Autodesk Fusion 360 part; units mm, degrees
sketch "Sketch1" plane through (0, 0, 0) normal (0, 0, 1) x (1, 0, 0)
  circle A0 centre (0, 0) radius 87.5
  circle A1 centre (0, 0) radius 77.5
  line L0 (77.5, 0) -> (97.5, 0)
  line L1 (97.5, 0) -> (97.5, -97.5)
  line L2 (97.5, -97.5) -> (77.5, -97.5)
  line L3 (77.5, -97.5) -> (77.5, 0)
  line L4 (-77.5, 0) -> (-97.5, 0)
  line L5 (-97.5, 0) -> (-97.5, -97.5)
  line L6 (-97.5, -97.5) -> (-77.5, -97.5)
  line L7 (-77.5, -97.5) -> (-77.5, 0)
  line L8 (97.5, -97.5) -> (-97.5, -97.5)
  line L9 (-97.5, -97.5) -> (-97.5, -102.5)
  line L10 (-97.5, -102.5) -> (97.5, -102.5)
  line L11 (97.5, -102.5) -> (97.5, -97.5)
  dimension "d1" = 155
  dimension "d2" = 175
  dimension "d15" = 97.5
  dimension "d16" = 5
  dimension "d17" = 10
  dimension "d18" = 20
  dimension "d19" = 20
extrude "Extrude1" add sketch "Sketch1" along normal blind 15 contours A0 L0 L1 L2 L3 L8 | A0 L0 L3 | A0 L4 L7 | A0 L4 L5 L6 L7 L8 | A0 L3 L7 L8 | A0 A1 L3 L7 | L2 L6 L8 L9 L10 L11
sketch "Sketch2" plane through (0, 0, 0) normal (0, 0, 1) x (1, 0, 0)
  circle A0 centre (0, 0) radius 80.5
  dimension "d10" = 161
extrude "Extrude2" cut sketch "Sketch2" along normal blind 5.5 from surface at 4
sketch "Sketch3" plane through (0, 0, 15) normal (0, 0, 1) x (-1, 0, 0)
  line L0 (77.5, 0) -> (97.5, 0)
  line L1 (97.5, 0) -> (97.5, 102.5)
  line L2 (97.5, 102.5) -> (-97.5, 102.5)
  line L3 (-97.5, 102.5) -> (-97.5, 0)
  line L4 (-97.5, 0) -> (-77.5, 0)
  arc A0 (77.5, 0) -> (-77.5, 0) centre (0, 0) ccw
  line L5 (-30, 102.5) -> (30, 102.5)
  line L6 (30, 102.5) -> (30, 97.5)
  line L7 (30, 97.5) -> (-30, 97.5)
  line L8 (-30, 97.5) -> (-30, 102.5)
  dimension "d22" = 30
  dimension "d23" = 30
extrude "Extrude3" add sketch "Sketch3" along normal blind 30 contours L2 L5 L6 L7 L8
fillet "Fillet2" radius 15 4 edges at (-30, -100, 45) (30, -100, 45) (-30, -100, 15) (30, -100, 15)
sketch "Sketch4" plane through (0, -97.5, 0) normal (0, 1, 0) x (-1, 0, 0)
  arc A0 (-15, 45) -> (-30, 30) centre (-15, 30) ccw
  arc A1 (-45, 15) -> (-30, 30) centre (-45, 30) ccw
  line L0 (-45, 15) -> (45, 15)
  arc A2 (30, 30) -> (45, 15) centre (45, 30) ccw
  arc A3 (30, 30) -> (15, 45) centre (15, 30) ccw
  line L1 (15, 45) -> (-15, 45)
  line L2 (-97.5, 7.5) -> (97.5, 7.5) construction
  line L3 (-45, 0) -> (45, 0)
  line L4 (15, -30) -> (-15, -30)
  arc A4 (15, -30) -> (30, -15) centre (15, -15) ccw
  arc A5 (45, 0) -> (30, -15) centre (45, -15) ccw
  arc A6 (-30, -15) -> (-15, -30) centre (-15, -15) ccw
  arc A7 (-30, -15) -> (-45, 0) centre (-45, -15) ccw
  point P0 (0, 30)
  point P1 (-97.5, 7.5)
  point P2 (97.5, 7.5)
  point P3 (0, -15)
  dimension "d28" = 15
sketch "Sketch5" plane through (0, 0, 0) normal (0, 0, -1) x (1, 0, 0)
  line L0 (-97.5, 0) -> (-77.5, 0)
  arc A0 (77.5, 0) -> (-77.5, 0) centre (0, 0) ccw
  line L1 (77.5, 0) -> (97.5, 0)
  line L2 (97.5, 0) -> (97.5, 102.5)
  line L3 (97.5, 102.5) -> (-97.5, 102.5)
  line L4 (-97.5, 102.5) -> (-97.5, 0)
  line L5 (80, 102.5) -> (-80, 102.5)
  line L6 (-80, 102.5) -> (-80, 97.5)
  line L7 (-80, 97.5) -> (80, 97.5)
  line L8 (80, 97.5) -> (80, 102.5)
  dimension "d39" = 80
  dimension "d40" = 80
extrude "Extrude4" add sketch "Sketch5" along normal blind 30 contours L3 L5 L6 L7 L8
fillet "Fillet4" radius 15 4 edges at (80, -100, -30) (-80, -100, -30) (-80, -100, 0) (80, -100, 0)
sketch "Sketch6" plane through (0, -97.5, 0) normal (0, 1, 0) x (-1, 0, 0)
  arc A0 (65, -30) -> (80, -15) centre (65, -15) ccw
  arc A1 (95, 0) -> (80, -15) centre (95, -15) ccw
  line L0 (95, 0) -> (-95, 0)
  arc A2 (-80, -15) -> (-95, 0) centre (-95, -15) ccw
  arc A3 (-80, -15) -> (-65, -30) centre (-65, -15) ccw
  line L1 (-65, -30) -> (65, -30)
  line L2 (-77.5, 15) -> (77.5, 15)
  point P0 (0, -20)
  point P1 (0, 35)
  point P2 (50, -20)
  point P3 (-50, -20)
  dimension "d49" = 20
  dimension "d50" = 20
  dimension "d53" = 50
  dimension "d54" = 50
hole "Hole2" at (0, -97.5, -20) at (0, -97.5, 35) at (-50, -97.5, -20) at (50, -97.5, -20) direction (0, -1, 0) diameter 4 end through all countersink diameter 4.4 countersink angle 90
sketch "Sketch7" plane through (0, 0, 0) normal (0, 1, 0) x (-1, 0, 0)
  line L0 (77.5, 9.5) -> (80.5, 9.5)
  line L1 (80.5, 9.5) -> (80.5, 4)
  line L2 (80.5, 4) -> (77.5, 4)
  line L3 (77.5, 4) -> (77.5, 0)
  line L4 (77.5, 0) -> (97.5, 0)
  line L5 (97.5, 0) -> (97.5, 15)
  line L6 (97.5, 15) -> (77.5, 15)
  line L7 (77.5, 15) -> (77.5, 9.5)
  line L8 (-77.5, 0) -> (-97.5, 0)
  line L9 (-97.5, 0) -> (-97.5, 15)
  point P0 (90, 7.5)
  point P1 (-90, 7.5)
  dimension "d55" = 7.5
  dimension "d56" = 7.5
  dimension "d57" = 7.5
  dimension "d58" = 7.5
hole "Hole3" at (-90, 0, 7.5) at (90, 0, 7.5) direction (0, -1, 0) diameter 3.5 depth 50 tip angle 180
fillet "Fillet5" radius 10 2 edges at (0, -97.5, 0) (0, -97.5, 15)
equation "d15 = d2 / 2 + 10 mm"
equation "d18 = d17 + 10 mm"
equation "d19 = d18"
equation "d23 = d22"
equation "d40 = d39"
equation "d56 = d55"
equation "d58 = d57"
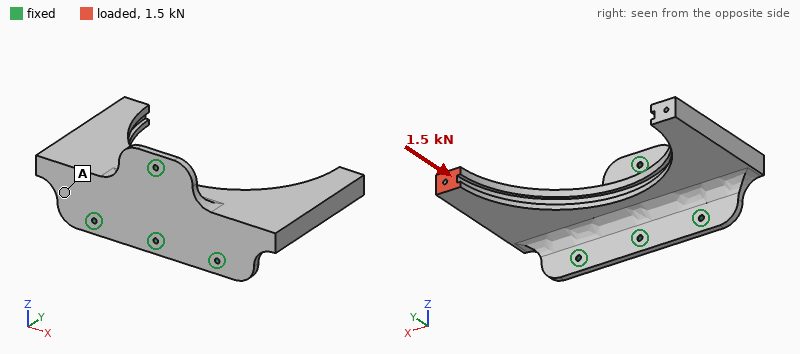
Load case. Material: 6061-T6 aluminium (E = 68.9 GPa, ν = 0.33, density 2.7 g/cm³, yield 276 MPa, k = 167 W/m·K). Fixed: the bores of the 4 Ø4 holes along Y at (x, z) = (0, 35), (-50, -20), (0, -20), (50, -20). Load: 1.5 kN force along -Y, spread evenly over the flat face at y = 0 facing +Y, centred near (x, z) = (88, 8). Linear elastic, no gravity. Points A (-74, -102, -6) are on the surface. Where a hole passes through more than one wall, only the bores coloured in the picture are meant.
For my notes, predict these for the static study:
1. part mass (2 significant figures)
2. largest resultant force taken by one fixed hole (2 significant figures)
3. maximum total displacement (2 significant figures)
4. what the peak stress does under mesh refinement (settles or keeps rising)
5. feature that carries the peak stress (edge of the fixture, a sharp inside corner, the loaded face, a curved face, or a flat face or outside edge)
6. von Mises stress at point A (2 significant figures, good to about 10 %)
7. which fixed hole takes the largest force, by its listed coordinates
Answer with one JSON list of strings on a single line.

["520 g", "1.7 kN", "0.39 mm", "keeps rising", "edge of the fixture", "9.8 MPa", "(50, -20)"]
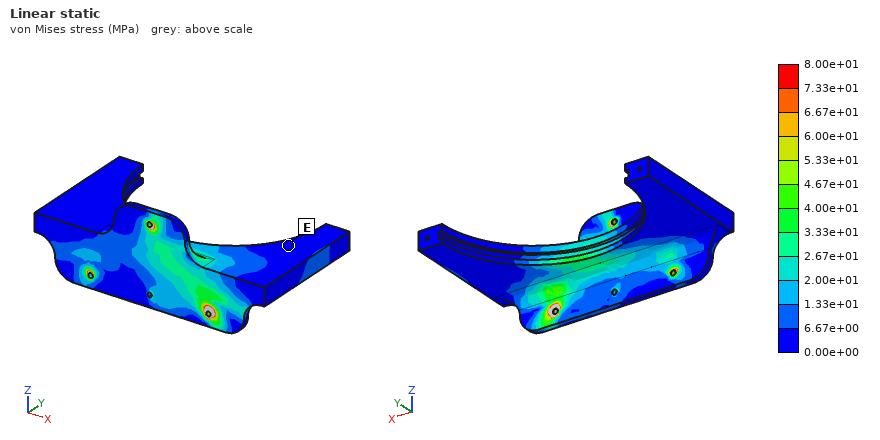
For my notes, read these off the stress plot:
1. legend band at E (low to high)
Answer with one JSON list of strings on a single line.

["0.00e+00 to 6.67e+00 MPa"]
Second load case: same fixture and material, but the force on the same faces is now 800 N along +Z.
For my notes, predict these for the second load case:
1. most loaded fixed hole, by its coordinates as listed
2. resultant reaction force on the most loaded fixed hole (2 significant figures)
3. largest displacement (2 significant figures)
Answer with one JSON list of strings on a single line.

["(0, 35)", "2.2 kN", "0.86 mm"]
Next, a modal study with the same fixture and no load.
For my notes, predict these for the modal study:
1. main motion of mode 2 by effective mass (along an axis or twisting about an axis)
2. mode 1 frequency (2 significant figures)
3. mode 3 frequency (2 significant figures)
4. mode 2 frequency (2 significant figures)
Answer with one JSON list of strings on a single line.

["along Z", "760 Hz", "1400 Hz", "860 Hz"]
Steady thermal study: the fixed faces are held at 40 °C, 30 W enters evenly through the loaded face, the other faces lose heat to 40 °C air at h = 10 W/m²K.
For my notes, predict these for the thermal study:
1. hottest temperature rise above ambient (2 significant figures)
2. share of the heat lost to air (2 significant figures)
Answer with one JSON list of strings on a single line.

["49 K", "12 %"]
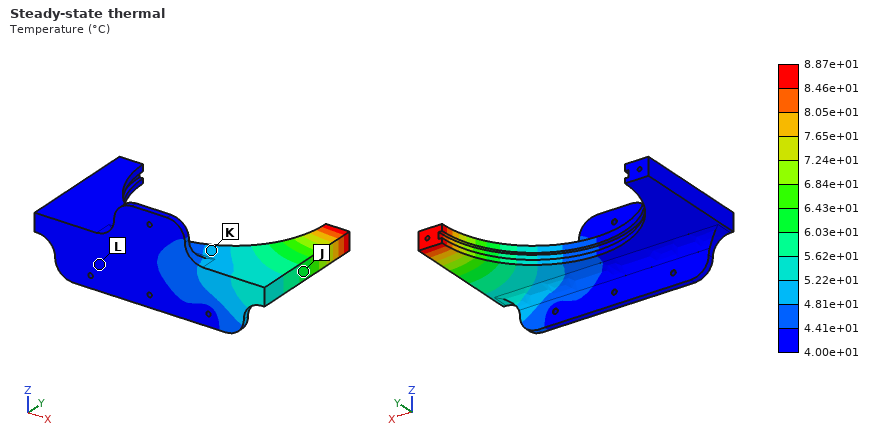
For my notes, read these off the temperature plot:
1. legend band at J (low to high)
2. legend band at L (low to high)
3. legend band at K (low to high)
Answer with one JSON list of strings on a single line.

["6.03e+01 to 6.43e+01 °C", "4.00e+01 to 4.41e+01 °C", "4.81e+01 to 5.22e+01 °C"]
